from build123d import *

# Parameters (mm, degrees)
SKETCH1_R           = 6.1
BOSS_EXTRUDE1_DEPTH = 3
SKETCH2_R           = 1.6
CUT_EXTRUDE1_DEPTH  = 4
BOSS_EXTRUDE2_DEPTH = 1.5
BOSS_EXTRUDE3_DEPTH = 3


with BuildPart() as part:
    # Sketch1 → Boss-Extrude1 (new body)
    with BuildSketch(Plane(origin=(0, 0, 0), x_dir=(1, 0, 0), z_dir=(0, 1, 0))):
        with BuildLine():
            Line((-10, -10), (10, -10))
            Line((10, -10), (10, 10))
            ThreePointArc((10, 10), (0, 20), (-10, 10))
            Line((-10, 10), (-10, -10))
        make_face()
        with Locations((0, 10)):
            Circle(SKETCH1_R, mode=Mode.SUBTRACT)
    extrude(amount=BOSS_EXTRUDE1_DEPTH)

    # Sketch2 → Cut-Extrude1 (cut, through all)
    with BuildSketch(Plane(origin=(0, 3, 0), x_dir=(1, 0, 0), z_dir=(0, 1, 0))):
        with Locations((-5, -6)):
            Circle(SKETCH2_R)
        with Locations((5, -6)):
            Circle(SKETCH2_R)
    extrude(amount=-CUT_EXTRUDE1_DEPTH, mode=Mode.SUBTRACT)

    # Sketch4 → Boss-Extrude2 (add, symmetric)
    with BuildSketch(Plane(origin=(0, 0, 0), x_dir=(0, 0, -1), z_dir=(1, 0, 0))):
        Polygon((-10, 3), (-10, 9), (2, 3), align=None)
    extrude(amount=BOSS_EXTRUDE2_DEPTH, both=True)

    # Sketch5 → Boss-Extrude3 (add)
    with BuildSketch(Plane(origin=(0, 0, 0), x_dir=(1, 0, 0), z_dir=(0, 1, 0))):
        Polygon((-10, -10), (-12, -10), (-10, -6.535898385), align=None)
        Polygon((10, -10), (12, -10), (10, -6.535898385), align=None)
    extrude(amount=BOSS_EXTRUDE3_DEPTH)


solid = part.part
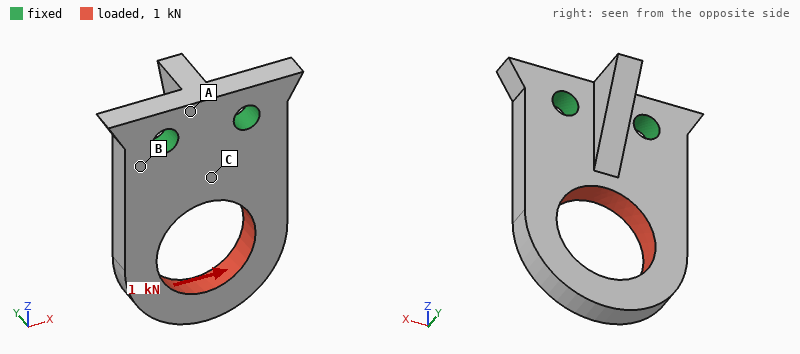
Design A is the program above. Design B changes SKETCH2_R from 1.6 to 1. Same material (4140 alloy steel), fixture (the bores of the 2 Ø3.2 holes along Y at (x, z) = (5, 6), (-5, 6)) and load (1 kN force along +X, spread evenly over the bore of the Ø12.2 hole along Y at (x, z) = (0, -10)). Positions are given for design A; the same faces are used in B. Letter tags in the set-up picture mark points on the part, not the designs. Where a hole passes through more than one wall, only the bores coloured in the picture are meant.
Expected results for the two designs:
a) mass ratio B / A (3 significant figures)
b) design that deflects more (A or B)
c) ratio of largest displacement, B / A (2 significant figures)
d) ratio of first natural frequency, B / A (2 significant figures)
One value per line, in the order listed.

1.02
B
1.1
0.94
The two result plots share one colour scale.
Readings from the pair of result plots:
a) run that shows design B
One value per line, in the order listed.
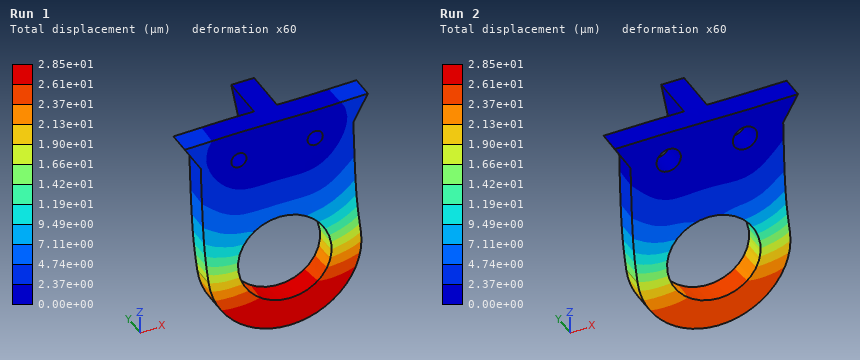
Run 1
